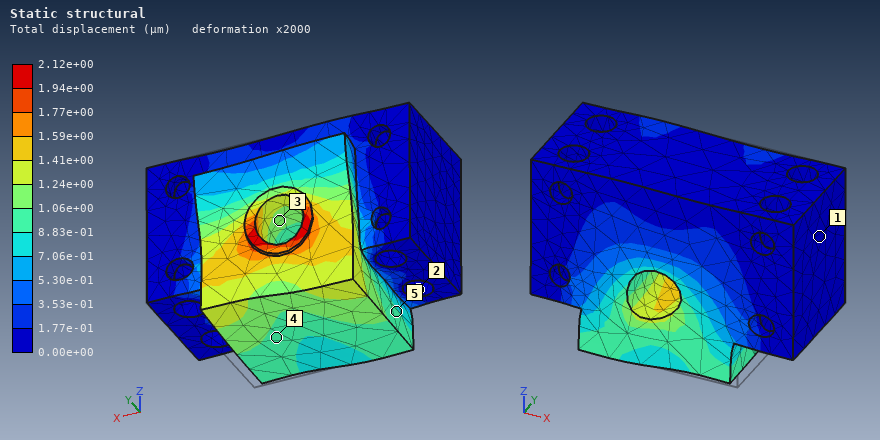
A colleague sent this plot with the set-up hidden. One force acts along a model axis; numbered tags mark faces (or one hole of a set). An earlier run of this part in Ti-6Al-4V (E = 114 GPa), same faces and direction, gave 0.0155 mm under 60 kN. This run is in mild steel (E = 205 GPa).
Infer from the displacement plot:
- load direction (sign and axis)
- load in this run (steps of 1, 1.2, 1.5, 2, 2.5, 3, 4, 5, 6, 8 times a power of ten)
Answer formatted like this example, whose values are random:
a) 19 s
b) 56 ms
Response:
a) -X
b) 15 kN
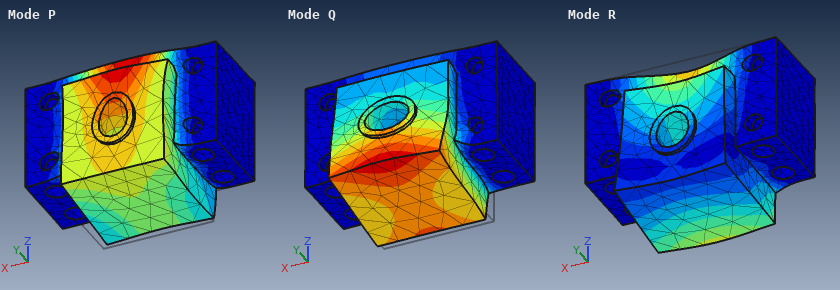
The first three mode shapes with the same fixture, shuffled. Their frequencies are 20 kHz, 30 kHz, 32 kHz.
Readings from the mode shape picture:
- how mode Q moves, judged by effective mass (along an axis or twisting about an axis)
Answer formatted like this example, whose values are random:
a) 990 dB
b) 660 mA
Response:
a) along Y
